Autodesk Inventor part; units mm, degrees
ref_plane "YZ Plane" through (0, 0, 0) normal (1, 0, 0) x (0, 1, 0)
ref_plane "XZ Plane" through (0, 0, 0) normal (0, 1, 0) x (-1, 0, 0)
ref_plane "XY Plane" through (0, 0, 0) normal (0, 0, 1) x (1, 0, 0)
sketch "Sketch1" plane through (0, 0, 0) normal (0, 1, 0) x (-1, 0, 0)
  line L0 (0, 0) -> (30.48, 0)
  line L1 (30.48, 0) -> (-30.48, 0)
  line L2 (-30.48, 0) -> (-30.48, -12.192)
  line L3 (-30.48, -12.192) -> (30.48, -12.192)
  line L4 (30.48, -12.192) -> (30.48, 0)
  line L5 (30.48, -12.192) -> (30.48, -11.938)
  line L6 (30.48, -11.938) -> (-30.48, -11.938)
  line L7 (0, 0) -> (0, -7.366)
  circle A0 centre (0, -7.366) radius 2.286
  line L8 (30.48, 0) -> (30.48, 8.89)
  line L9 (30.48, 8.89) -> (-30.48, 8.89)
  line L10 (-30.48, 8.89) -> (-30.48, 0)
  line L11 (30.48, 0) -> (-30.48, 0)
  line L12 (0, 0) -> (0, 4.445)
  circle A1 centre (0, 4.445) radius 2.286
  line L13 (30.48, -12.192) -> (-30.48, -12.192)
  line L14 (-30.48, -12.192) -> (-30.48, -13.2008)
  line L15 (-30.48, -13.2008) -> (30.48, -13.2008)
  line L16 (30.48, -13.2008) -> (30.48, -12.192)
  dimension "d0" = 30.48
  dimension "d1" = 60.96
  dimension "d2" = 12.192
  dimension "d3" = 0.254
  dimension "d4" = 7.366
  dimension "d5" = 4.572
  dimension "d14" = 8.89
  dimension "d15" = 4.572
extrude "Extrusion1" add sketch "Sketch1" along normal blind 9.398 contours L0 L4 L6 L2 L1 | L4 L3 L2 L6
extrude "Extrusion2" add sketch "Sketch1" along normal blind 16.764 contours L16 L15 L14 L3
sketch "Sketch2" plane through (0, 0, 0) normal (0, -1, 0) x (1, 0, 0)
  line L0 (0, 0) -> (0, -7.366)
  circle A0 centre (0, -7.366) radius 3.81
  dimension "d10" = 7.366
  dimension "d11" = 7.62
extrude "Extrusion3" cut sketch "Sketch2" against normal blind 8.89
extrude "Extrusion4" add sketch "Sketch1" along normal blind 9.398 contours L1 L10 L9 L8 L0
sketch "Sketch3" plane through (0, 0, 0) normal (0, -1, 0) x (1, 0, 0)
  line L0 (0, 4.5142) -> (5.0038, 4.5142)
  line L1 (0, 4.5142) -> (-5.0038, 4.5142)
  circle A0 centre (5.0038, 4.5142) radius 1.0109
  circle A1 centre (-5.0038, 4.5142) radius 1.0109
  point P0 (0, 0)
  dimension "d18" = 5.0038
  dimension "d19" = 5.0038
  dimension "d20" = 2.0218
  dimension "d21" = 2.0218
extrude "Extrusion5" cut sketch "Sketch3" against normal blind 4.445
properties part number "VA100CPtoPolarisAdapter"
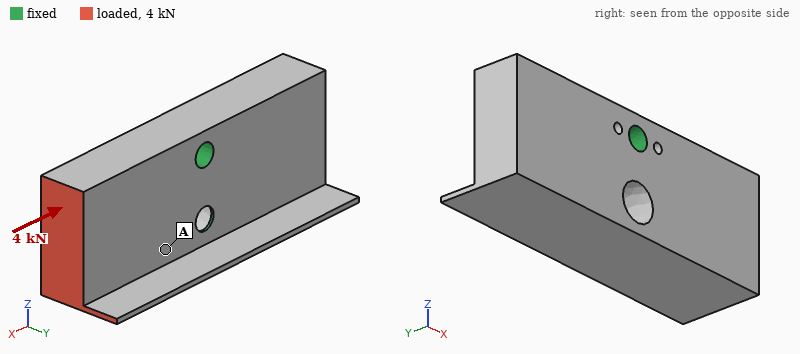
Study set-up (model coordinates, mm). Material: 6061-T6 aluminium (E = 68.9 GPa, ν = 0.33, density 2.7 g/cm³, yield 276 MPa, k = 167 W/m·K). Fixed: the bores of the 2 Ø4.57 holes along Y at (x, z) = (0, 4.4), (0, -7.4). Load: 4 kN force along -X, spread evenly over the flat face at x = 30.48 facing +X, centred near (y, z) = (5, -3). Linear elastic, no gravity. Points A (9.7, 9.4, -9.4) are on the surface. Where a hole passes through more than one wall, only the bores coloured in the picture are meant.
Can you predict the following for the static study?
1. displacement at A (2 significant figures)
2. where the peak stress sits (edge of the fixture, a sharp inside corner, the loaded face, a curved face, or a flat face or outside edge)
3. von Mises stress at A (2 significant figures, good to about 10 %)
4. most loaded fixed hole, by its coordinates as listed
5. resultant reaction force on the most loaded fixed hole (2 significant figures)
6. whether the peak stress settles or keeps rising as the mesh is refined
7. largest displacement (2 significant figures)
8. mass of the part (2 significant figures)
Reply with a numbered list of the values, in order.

1. 16 µm
2. edge of the fixture
3. 25 MPa
4. (0, 4.4)
5. 2.5 kN
6. keeps rising
7. 40 µm
8. 34 g
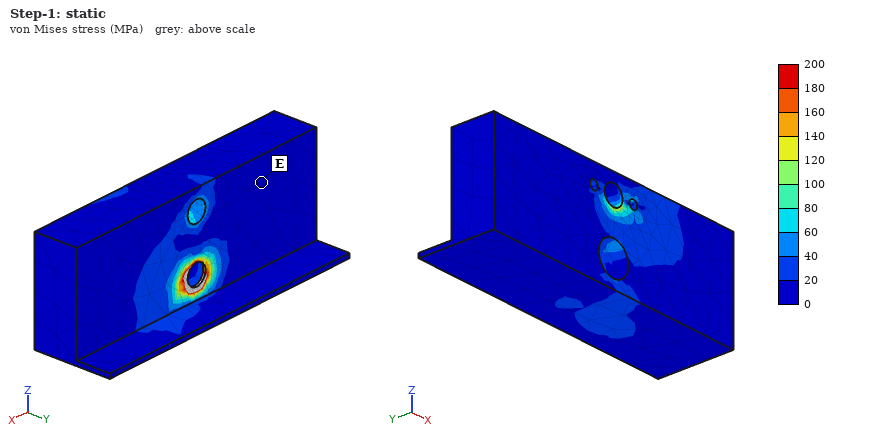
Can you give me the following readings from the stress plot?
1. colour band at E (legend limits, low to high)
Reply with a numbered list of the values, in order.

1. 0 to 20 MPa
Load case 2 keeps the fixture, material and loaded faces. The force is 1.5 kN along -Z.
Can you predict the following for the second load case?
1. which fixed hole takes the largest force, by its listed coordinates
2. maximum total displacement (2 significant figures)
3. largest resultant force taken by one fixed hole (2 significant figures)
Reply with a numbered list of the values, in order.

1. (0, 4.4)
2. 0.17 mm
3. 2.5 kN
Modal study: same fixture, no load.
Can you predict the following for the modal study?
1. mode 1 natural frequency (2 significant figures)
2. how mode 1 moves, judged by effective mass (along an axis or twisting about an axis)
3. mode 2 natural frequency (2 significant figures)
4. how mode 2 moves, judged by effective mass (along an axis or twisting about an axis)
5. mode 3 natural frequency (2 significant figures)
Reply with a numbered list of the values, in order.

1. 5500 Hz
2. twisting about Z
3. 7800 Hz
4. along Y
5. 8100 Hz
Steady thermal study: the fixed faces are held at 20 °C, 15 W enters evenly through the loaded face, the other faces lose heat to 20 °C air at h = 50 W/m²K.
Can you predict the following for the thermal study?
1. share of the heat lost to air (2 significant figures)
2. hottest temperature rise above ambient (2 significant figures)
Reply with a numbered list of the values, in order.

1. 6.9 %
2. 14 K
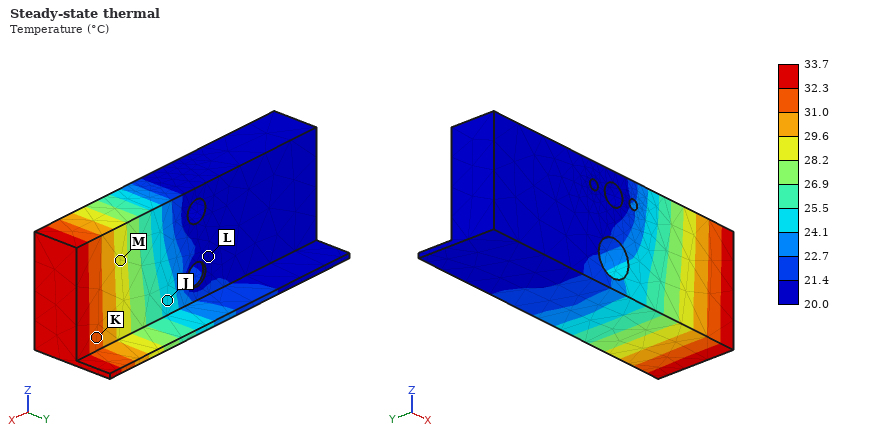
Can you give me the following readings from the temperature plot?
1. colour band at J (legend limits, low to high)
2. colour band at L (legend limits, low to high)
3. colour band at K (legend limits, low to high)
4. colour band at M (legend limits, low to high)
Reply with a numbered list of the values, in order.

1. 24.1 to 25.5 °C
2. 20.0 to 21.4 °C
3. 31.0 to 32.3 °C
4. 28.2 to 29.6 °C
